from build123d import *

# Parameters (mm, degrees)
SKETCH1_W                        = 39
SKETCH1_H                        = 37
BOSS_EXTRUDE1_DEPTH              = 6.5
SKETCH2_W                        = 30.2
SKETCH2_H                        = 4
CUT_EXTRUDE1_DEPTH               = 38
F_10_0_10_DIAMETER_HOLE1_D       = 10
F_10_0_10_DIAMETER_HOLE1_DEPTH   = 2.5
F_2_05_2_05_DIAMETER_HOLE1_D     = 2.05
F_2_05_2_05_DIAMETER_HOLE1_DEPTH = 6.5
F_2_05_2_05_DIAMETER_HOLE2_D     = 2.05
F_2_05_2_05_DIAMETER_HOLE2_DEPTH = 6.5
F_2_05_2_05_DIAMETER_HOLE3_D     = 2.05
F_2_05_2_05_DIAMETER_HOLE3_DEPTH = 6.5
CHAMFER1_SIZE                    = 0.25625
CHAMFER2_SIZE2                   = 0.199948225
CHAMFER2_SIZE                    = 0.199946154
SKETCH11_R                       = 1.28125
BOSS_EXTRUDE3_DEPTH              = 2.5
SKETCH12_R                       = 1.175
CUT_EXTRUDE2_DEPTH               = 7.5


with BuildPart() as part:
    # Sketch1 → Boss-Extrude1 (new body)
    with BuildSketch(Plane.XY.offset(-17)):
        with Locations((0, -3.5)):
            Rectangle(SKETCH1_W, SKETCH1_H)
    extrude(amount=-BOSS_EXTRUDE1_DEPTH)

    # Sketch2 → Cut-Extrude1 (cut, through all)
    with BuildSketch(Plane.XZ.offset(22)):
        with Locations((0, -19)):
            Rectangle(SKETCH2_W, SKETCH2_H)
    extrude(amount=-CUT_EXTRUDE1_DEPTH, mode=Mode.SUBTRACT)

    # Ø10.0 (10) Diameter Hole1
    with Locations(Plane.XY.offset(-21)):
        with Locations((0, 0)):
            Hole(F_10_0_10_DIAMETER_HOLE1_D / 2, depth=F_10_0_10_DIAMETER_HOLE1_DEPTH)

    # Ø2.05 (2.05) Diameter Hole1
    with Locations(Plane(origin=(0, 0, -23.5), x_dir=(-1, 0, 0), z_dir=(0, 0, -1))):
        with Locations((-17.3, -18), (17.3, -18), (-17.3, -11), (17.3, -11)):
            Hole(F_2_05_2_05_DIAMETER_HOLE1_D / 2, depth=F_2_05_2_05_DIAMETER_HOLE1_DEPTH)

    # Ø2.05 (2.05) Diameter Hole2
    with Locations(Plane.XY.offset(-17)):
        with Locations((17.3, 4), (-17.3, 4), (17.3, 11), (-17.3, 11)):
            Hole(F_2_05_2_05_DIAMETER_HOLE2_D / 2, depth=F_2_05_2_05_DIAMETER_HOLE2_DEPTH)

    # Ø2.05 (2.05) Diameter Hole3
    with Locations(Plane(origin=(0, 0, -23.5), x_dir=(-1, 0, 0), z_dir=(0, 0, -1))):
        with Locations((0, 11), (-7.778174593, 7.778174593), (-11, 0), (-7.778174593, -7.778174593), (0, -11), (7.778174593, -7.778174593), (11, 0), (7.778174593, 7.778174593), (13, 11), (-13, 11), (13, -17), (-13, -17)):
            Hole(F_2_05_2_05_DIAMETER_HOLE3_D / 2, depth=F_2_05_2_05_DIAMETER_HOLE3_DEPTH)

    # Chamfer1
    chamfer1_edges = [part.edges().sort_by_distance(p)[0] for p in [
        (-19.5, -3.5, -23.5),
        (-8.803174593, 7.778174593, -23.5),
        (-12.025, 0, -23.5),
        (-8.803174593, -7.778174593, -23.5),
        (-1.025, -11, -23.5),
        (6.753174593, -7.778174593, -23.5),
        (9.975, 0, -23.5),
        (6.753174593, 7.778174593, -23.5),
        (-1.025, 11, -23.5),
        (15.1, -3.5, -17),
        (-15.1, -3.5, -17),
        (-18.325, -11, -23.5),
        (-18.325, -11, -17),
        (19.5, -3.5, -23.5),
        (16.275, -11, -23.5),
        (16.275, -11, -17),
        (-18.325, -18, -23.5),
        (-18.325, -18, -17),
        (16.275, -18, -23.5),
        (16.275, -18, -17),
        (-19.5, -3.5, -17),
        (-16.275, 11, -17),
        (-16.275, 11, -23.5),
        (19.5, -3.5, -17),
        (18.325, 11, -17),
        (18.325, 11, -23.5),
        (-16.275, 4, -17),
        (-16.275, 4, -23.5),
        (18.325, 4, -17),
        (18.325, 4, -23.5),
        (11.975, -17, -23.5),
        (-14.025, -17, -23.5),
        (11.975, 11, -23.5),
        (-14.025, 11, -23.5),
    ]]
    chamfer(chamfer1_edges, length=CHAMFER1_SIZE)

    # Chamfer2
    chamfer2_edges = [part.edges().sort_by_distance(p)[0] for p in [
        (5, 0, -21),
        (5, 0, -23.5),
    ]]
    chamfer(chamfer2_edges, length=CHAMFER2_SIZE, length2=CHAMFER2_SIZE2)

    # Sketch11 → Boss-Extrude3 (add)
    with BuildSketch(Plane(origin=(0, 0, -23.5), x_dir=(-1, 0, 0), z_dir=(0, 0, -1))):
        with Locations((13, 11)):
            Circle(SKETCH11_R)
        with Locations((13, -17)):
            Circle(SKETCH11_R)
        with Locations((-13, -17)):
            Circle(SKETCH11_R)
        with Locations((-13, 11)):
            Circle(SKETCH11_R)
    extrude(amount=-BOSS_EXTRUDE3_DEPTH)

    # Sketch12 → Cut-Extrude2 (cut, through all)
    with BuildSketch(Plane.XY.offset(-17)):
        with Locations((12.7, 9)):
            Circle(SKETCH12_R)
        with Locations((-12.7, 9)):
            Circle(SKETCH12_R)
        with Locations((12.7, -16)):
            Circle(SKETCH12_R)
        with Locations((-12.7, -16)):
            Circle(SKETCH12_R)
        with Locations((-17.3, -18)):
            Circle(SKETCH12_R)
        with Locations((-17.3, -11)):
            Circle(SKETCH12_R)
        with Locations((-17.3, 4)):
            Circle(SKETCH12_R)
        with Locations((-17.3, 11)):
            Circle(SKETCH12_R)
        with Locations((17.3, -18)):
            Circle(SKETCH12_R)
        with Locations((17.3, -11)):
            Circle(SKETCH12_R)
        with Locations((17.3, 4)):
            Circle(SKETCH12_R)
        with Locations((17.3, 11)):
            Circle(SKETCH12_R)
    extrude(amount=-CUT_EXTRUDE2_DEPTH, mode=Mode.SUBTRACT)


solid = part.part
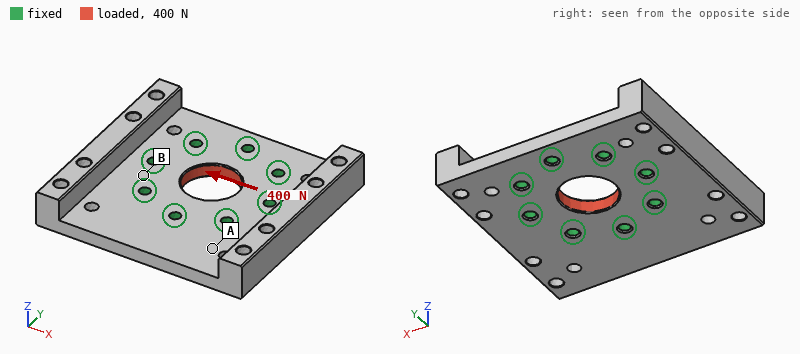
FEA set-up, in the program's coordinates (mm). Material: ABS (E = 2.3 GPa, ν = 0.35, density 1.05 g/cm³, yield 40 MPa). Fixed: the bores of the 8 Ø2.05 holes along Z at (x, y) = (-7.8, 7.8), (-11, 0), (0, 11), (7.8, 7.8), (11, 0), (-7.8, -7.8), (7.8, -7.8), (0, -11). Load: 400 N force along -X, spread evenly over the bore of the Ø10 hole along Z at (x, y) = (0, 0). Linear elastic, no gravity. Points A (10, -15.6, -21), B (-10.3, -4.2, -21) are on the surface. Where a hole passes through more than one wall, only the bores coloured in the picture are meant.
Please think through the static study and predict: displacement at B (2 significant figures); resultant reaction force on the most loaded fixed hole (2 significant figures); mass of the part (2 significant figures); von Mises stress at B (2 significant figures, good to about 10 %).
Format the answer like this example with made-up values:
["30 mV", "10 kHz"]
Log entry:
["4.4 µm", "78 N", "4.6 g", "1.8 MPa"]
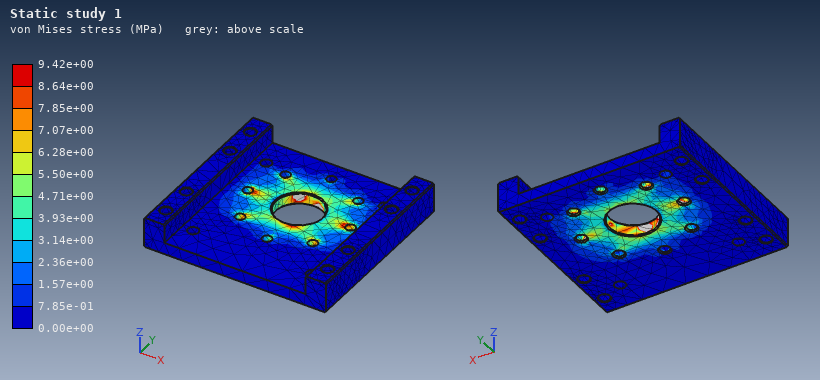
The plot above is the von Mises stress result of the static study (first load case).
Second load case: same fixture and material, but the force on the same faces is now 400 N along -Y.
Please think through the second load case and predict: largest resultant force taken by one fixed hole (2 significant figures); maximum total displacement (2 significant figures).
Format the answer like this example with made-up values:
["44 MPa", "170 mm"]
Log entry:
["79 N", "16 µm"]
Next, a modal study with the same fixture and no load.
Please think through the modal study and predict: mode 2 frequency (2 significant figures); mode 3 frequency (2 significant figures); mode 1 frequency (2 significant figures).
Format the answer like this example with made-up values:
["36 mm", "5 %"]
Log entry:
["2600 Hz", "3600 Hz", "2500 Hz"]
